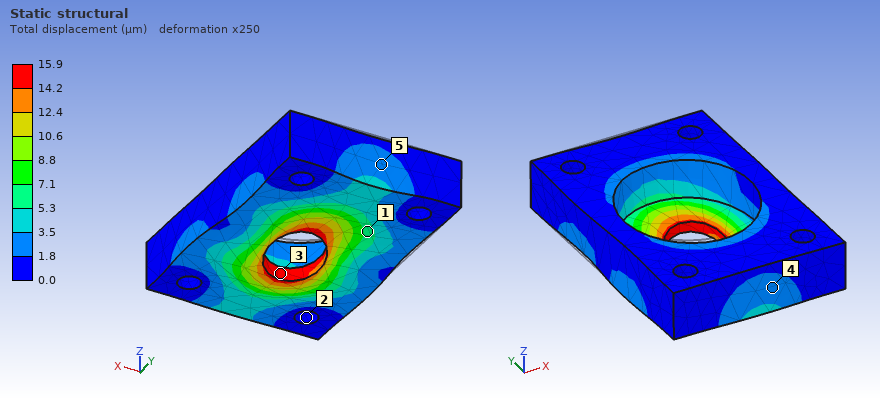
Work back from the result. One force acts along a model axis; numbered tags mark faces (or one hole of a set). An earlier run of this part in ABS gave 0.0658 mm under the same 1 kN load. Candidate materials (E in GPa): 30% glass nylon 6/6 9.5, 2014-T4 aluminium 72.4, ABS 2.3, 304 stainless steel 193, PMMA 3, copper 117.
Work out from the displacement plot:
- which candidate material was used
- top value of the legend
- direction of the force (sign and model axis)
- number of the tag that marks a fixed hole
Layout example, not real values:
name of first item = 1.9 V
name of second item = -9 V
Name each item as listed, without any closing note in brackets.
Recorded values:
which candidate material was used = 30% glass nylon 6/6
top value of the legend = 15.9 µm
direction of the force = -Y
number of the tag that marks a fixed hole = 2
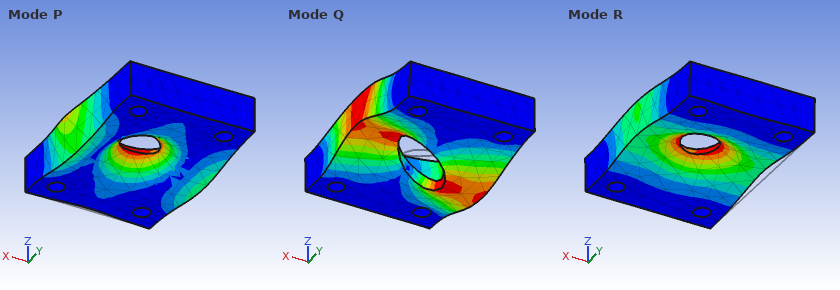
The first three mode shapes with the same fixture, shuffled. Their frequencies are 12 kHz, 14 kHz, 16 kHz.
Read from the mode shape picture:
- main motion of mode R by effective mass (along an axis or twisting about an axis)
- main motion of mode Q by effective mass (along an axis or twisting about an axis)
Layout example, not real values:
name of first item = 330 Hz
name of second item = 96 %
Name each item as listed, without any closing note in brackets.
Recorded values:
main motion of mode R by effective mass = along Z
main motion of mode Q by effective mass = twisting about Y
